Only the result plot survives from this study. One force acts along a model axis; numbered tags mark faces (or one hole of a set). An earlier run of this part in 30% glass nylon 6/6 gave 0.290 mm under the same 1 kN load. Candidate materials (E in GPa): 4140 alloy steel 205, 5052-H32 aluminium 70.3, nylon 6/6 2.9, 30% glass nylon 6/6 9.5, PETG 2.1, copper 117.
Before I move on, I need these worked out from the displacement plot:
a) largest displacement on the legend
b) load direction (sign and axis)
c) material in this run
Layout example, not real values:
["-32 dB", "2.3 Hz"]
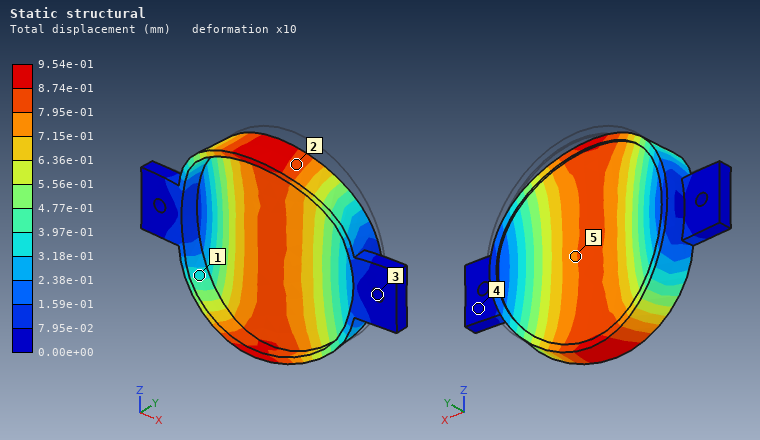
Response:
["9.54e-01 mm", "-Y", "nylon 6/6"]
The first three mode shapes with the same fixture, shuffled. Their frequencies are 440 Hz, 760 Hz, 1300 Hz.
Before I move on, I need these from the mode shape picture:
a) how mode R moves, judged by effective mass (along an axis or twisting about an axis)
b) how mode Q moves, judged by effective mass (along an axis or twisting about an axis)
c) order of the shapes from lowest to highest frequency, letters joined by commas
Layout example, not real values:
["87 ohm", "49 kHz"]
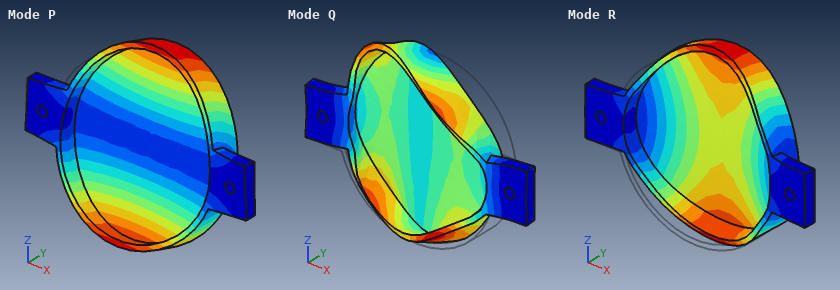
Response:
["along Y", "along X", "P, R, Q"]
